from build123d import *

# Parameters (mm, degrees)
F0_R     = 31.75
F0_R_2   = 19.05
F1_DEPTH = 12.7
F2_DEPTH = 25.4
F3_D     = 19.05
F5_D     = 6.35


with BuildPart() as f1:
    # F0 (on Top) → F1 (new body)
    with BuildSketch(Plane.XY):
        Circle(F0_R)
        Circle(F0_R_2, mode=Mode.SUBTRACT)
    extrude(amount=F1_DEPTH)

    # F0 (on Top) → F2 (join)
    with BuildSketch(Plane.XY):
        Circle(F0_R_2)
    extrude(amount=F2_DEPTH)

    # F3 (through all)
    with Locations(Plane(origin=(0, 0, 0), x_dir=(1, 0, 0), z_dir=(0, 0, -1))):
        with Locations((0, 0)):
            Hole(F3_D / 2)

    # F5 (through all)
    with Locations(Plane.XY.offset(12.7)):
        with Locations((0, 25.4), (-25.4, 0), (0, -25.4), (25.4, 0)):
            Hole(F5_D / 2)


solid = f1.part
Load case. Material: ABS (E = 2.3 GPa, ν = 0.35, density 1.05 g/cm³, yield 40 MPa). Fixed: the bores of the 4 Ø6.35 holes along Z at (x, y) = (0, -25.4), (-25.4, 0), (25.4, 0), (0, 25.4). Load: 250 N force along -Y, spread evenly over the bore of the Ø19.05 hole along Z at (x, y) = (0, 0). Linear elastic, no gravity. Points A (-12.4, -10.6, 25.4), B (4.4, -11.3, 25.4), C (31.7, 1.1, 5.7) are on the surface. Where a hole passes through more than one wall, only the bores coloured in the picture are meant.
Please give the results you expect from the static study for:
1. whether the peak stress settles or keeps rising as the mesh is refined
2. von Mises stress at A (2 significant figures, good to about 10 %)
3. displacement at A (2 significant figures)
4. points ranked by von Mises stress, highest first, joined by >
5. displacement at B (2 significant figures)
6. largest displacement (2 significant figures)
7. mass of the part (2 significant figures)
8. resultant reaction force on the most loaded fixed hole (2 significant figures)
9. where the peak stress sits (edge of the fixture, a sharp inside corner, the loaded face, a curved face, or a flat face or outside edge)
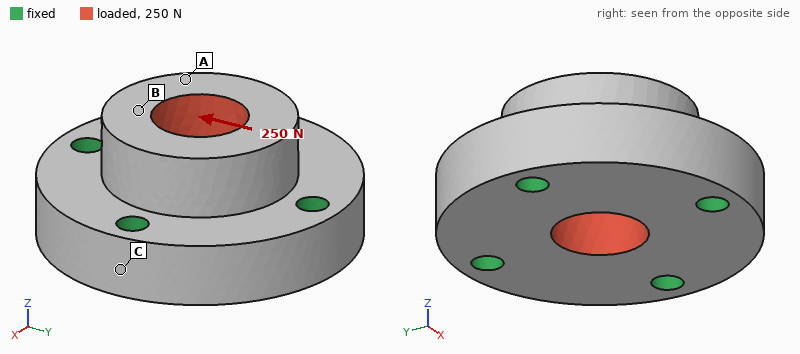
keeps rising
0.16 MPa
4.9 µm
B > A > C
5.7 µm
6.1 µm
48 g
83 N
a sharp inside corner
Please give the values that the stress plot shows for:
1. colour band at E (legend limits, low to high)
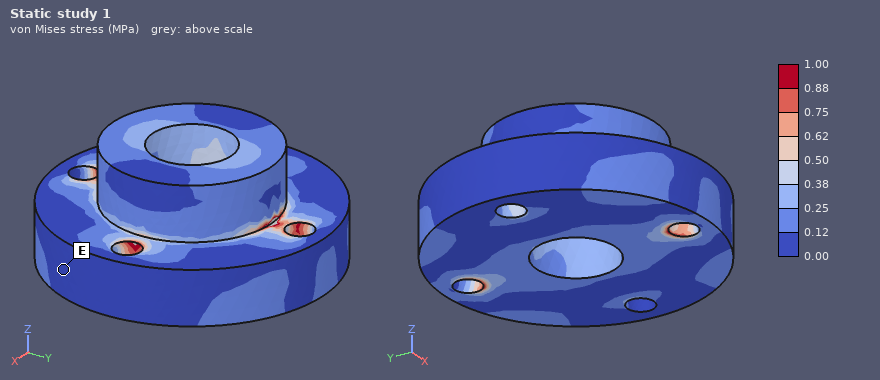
0.00 to 0.12 MPa
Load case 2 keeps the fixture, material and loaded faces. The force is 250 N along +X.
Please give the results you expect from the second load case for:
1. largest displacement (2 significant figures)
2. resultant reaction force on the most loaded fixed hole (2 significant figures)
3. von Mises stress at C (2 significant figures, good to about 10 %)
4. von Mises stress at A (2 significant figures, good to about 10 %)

6.1 µm
83 N
0.15 MPa
0.18 MPa
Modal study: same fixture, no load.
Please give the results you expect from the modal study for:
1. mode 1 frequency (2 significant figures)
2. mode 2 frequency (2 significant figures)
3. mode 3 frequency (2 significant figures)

7400 Hz
7400 Hz
7500 Hz
